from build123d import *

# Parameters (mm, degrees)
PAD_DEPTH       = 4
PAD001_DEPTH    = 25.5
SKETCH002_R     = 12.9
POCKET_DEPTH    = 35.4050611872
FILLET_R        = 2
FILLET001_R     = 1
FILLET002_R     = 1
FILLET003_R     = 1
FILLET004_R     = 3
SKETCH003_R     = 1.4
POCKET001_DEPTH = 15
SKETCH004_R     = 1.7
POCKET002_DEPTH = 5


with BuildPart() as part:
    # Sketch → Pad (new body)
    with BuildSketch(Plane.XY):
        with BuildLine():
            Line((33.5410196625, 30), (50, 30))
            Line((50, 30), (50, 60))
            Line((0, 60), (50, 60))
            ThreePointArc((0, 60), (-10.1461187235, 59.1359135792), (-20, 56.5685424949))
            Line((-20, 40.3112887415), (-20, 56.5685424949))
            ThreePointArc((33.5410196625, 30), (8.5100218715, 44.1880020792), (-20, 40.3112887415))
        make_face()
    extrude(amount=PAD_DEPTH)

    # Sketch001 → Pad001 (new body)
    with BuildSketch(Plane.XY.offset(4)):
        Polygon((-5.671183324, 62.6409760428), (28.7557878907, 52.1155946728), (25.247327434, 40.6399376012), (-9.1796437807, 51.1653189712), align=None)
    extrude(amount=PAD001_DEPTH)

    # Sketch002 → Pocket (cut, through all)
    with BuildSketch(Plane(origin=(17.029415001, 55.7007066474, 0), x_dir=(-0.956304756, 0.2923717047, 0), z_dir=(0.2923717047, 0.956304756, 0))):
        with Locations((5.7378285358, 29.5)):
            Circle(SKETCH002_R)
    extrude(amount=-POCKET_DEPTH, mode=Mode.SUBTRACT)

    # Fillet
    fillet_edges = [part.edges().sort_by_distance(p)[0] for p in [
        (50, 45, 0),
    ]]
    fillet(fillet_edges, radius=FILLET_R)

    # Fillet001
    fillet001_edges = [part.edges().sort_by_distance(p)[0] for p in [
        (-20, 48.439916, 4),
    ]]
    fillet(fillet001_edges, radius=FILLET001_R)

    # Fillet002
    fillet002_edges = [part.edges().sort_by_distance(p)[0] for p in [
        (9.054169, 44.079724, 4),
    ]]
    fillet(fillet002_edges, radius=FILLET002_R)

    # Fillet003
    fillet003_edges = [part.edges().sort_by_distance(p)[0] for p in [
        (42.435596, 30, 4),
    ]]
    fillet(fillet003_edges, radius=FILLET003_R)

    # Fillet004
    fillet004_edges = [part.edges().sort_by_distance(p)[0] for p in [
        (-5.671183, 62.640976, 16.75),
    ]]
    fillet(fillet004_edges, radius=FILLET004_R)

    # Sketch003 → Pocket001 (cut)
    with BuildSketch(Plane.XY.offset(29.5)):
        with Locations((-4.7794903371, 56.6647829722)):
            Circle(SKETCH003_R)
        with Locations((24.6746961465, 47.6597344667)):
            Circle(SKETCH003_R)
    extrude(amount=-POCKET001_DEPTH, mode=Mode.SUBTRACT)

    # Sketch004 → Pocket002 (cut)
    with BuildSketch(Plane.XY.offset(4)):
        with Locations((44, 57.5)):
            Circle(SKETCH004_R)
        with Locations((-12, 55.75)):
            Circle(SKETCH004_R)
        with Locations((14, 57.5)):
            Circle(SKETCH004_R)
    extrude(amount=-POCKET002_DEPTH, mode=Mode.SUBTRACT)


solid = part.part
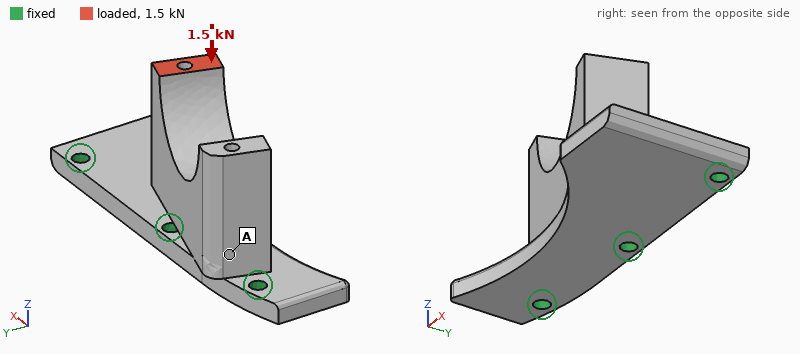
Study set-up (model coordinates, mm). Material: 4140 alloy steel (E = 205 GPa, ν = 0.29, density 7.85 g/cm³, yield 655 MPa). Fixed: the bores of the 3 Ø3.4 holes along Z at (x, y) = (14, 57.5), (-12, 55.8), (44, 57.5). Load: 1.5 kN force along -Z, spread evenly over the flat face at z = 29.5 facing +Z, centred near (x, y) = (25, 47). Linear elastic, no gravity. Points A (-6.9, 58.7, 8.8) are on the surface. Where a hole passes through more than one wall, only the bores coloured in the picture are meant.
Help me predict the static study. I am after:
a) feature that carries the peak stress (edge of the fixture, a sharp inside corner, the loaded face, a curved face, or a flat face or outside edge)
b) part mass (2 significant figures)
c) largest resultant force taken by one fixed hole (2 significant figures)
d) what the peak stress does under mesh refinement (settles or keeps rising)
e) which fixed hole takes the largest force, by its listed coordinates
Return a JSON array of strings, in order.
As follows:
["edge of the fixture", "100 g", "1.6 kN", "keeps rising", "(14, 57.5)"]
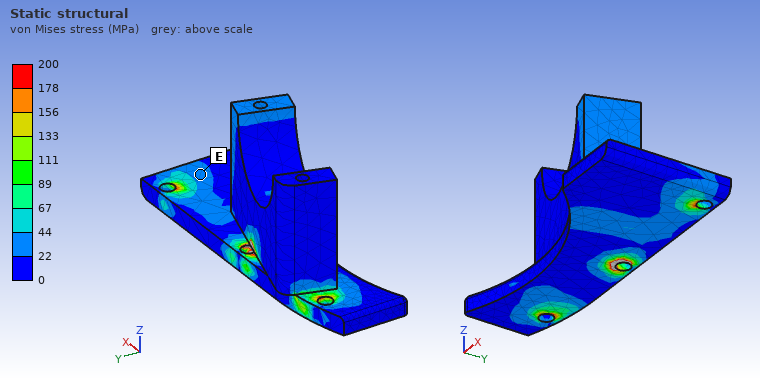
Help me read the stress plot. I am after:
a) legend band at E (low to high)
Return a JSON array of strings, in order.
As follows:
["22 to 44 MPa"]
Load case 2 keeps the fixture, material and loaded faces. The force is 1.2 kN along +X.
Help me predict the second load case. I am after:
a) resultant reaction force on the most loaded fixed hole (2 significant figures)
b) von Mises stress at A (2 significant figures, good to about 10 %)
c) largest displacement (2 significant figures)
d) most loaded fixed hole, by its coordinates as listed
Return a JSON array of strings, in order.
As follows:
["1.4 kN", "9.2 MPa", "30 µm", "(-12, 55.8)"]
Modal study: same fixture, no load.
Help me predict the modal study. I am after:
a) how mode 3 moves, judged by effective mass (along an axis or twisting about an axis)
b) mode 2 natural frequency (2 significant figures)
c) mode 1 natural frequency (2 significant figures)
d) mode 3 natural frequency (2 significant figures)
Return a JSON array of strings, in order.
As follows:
["along X", "7300 Hz", "3900 Hz", "12 kHz"]
